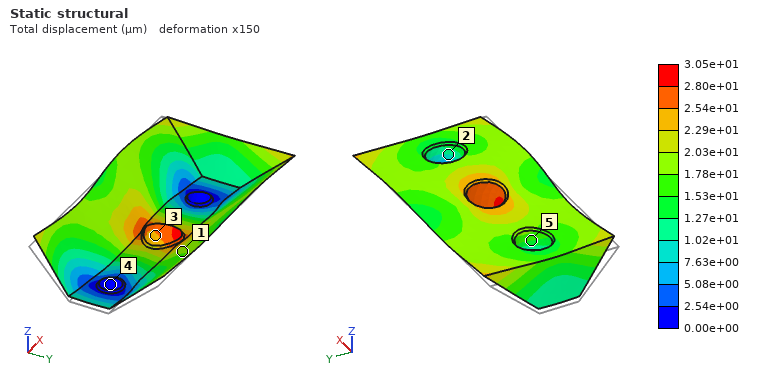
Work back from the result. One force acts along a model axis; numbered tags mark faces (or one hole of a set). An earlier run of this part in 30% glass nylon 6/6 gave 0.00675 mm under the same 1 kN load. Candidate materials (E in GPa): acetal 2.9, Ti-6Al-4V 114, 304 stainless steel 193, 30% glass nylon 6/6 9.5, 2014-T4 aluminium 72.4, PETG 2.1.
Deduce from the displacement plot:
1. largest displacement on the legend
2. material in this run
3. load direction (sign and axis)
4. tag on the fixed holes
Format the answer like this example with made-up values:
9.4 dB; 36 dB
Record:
3.05e+01 µm; PETG; +X; 4
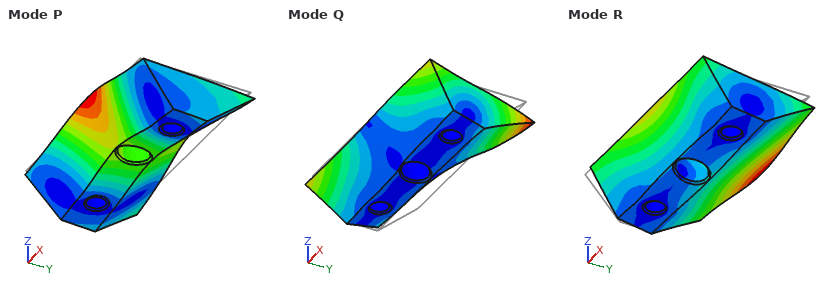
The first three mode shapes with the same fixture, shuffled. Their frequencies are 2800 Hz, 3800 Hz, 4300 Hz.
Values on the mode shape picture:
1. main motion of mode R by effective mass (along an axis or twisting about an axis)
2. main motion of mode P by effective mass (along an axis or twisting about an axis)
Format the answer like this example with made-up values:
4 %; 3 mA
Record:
along Y; along Z
